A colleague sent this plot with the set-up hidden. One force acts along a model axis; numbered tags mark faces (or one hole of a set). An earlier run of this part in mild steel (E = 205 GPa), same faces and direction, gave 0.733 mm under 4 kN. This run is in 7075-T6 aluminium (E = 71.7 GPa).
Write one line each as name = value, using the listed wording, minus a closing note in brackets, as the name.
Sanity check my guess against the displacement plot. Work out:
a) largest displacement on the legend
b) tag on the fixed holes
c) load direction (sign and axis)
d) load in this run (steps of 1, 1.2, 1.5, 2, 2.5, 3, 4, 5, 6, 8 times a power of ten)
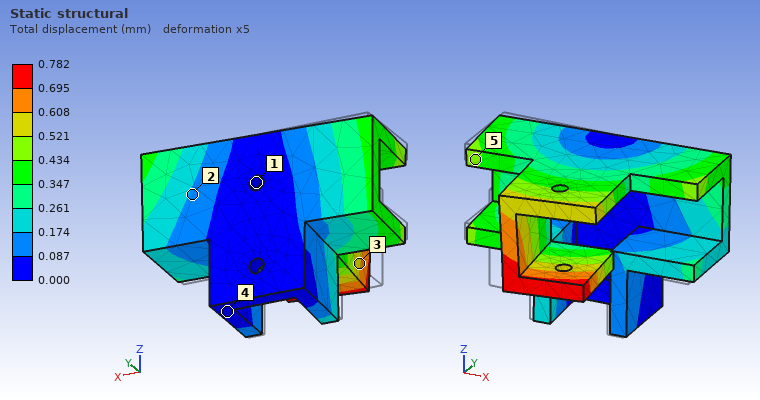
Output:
largest displacement on the legend = 0.782 mm
tag on the fixed holes = 1
load direction = +X
load in this run = 1.5 kN
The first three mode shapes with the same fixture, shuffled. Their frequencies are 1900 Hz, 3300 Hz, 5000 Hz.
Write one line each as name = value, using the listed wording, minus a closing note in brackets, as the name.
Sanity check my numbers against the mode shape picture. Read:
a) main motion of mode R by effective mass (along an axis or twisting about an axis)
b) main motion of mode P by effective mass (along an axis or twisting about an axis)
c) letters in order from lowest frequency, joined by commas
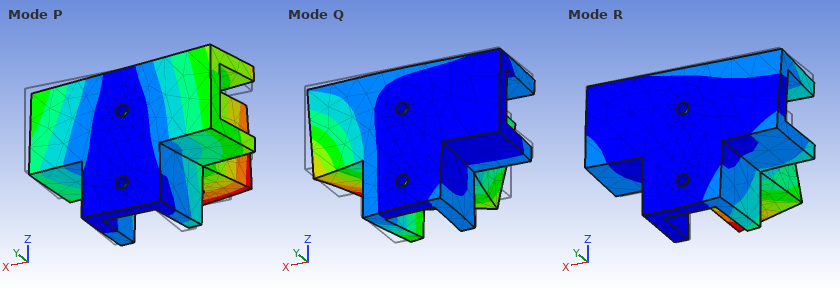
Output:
main motion of mode R by effective mass = along Z
main motion of mode P by effective mass = along X
letters in order from lowest frequency, joined by commas = P, R, Q
